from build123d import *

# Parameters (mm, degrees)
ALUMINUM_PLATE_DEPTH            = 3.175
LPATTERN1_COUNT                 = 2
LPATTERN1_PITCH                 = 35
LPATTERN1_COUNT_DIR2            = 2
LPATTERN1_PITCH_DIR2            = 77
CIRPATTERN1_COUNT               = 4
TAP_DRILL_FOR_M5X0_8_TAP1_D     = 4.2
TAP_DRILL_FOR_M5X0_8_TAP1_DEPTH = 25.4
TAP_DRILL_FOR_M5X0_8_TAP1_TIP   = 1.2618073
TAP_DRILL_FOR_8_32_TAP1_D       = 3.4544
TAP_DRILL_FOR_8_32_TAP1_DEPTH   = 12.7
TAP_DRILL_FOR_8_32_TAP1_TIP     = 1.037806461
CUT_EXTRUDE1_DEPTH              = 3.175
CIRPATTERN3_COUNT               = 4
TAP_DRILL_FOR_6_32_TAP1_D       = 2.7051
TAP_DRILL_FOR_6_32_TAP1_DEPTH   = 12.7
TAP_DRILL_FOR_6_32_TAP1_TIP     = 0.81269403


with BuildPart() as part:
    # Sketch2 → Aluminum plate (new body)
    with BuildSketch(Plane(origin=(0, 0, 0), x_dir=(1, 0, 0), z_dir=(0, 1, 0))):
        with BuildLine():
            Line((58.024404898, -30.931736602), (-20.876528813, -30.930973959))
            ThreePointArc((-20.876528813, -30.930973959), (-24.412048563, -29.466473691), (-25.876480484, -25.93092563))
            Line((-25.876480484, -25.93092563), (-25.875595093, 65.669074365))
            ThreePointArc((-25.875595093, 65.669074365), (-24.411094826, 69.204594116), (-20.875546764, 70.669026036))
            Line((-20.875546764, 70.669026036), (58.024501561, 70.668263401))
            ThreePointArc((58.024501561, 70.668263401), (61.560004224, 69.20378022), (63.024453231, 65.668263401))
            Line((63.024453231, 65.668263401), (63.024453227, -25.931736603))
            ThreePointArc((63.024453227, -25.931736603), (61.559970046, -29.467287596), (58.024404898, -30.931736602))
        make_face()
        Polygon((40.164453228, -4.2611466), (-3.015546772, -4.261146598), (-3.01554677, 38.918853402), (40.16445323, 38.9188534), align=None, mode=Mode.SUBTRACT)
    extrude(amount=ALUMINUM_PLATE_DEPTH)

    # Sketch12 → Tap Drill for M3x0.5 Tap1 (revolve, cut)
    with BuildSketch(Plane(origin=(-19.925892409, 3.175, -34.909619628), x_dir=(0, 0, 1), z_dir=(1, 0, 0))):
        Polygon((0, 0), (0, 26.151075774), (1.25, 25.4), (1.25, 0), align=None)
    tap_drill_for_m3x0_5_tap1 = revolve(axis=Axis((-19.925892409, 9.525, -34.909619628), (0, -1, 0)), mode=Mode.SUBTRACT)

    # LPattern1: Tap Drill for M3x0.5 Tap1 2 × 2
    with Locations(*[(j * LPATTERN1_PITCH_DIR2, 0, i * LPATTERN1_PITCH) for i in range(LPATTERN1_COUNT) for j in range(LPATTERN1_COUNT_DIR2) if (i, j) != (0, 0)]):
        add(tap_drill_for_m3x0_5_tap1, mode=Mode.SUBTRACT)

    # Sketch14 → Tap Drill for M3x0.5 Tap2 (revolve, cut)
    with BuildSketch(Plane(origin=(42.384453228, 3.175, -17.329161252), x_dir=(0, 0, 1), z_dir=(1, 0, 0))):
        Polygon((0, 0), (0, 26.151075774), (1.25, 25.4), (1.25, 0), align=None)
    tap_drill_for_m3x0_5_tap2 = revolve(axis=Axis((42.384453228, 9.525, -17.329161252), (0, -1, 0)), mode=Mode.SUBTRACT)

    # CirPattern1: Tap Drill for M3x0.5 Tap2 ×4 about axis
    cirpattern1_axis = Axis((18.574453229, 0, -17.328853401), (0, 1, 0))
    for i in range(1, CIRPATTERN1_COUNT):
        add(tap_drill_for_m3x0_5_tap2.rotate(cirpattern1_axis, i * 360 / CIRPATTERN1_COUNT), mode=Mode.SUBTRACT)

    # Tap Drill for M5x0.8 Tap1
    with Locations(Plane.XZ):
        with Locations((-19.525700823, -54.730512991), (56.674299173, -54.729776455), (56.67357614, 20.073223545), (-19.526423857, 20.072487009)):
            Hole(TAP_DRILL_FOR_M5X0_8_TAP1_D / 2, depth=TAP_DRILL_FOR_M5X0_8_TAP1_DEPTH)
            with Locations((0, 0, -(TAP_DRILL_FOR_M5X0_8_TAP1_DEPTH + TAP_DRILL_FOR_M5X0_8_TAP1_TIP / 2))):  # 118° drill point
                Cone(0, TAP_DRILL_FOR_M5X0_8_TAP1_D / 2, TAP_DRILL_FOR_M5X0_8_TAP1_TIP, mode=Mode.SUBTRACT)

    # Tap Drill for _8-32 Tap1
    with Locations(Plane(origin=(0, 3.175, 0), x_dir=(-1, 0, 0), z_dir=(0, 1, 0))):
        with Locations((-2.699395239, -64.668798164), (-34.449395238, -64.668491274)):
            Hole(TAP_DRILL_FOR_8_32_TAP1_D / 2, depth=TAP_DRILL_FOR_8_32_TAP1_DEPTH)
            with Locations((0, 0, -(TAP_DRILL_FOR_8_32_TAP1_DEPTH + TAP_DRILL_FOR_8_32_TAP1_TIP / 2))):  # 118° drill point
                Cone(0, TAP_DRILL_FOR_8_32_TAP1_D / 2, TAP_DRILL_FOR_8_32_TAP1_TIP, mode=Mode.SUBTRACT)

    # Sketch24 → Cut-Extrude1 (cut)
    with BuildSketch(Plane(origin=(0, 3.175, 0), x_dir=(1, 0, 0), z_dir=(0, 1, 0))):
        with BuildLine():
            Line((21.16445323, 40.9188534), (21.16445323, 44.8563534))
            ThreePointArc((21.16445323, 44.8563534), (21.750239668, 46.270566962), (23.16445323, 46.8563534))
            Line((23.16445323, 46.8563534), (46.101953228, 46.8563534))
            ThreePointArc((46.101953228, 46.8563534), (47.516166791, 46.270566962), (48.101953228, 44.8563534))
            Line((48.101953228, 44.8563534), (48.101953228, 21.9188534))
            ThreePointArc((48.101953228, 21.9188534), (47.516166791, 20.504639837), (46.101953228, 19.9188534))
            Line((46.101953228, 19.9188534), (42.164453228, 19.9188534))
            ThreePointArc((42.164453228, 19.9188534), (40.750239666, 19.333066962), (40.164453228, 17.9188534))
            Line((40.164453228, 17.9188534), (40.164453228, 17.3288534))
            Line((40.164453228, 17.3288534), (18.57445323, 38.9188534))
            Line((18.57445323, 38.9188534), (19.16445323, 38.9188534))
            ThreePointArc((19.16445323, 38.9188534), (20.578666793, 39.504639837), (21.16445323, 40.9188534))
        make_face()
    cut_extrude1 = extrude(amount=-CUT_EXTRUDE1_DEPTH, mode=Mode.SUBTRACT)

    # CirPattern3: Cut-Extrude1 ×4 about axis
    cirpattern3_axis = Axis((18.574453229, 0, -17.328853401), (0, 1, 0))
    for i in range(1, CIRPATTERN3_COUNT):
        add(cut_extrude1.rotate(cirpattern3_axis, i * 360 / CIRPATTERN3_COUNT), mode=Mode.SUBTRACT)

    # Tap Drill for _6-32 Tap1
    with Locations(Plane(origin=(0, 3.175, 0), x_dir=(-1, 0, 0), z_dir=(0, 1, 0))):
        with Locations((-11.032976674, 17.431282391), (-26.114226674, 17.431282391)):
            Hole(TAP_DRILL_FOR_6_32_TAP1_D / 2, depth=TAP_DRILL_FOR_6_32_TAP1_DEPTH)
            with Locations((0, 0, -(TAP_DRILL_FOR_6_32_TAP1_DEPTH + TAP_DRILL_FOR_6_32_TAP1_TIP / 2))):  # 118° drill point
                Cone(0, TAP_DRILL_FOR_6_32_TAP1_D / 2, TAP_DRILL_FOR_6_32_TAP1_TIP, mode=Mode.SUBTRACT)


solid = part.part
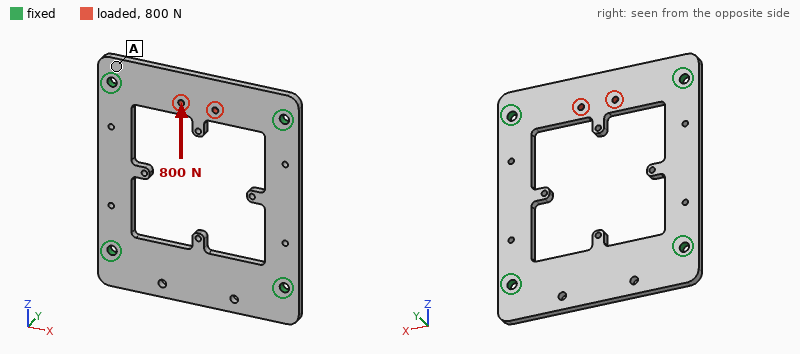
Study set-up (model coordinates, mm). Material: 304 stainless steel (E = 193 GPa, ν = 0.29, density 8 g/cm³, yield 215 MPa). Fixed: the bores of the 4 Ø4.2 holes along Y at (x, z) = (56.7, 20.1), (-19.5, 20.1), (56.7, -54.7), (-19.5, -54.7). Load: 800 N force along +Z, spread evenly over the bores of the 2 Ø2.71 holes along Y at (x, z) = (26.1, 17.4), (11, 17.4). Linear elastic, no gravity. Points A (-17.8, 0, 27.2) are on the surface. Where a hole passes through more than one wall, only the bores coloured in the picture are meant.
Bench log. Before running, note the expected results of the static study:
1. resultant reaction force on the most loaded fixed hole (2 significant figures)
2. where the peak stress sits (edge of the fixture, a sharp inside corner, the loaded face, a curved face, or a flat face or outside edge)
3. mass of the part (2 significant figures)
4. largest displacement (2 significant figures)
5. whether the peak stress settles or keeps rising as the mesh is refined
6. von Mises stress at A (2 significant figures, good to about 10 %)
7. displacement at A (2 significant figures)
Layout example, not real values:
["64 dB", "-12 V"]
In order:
["340 N", "edge of the fixture", "140 g", "11 µm", "keeps rising", "8.8 MPa", "1.7 µm"]
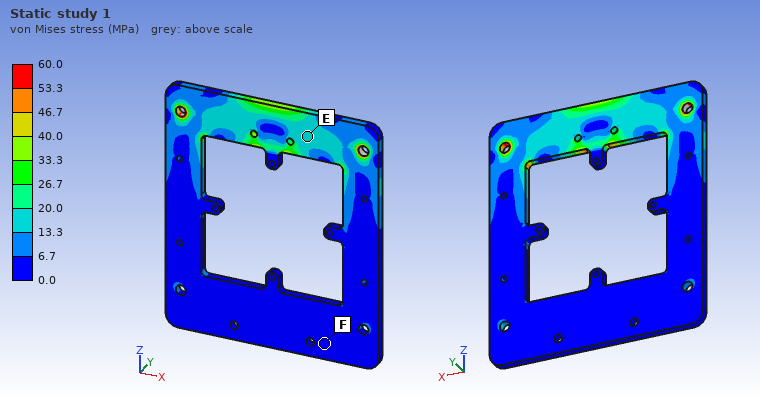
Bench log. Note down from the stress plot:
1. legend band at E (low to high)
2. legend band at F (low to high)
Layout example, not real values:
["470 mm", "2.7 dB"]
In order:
["13.3 to 20.0 MPa", "0.0 to 6.7 MPa"]
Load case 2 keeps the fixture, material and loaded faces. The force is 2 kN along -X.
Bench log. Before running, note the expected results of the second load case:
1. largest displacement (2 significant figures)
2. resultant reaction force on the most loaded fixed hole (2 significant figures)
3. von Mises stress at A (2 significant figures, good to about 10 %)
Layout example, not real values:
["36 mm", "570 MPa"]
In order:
["4.8 µm", "1.0 kN", "8.2 MPa"]
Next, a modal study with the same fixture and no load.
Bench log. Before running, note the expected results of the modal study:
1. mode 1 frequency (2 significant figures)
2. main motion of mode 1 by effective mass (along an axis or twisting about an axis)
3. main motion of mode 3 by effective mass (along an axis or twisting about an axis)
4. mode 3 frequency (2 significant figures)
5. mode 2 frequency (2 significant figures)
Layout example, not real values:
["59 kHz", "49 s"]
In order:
["2600 Hz", "along Y", "along Y", "2900 Hz", "2800 Hz"]
